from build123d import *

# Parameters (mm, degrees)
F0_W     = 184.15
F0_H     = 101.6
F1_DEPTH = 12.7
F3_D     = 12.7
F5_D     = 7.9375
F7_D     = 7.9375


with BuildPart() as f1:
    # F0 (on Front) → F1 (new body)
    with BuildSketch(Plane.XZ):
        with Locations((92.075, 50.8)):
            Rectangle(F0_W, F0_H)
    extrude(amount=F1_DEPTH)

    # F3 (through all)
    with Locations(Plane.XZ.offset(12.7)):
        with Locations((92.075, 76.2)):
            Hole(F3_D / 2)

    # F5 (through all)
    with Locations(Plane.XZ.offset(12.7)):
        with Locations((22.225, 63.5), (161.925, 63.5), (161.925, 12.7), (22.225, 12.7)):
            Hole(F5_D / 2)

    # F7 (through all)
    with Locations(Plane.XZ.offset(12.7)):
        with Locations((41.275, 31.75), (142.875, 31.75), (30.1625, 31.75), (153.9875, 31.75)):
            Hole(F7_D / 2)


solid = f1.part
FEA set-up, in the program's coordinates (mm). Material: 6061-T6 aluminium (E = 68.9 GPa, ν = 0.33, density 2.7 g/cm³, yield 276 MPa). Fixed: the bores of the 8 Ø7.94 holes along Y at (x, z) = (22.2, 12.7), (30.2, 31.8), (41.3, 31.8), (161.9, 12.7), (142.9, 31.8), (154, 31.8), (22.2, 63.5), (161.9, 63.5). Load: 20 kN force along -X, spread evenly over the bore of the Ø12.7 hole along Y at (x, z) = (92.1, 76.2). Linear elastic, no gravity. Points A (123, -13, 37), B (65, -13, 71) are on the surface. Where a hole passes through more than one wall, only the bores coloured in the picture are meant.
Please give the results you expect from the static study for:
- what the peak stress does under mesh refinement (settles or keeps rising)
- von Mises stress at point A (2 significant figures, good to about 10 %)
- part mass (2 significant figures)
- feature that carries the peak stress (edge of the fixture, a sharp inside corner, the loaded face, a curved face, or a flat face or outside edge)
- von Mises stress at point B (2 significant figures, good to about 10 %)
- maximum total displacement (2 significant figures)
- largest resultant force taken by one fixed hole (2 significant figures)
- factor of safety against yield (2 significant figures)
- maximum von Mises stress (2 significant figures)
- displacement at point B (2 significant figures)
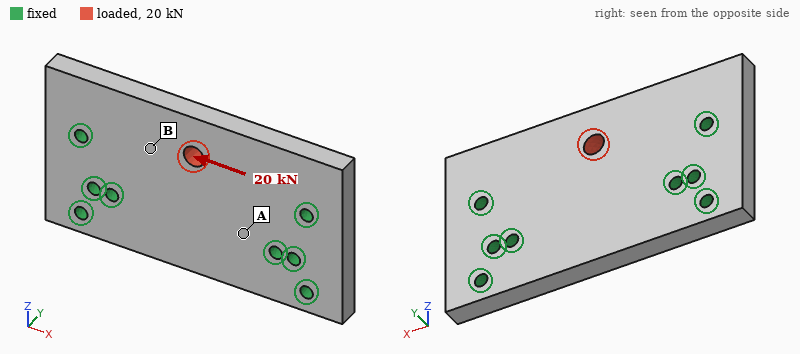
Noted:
settles
9.5 MPa
620 g
the loaded face
21 MPa
22 µm
6.5 kN
4.0
69 MPa
11 µm
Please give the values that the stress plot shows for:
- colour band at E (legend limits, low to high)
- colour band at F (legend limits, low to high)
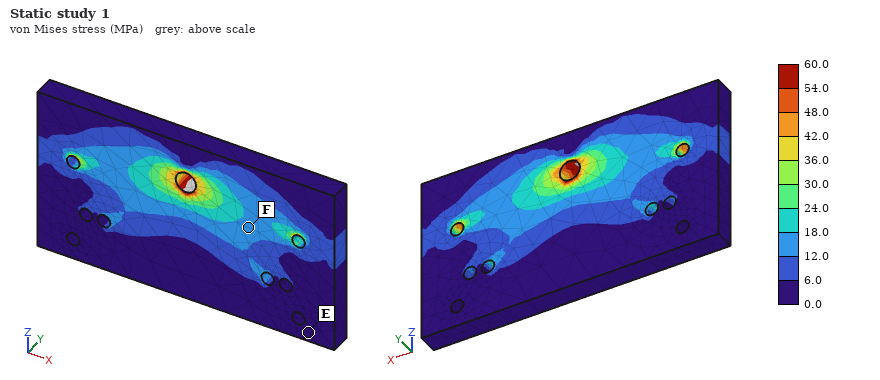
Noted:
0.0 to 6.0 MPa
12.0 to 18.0 MPa
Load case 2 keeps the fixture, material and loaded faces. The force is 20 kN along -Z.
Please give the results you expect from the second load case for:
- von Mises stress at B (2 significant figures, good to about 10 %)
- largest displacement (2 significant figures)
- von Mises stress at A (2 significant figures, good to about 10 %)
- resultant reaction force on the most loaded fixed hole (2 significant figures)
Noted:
17 MPa
35 µm
19 MPa
7.4 kN
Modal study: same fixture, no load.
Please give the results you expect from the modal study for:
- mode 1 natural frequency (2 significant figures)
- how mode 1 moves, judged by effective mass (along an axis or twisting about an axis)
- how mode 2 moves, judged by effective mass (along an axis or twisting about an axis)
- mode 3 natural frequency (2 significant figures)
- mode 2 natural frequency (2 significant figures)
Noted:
3100 Hz
along Y
along Y
6000 Hz
5300 Hz
